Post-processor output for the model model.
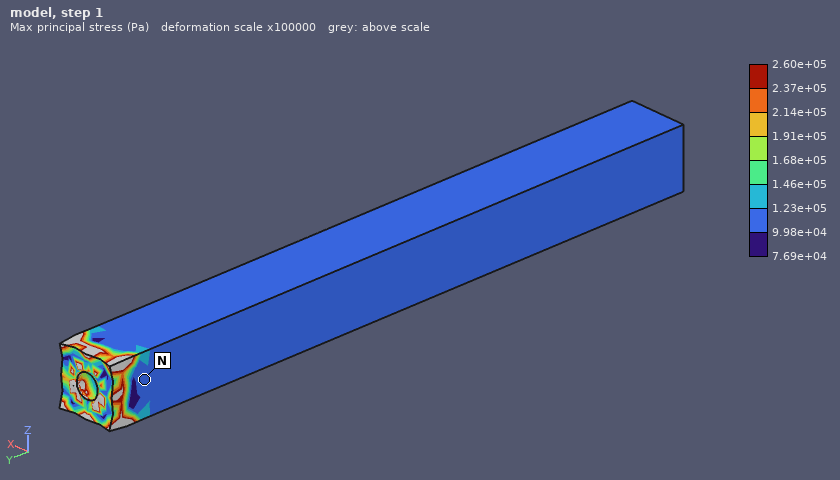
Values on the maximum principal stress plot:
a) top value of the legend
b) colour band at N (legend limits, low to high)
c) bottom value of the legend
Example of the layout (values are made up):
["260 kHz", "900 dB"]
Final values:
["2.60e+05 Pa", "9.98e+04 to 1.23e+05 Pa", "7.69e+04 Pa"]
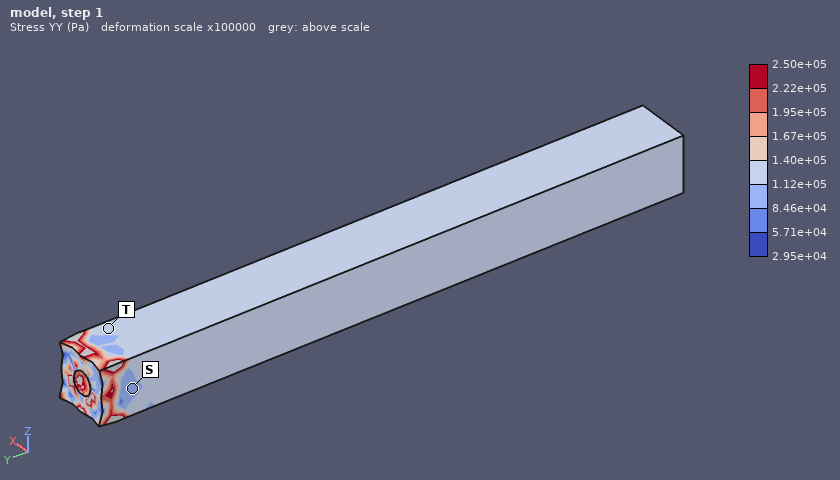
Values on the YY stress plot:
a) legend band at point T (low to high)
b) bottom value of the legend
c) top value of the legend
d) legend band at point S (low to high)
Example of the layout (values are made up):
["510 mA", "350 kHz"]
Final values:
["1.12e+05 to 1.40e+05 Pa", "2.95e+04 Pa", "2.50e+05 Pa", "8.46e+04 to 1.12e+05 Pa"]
